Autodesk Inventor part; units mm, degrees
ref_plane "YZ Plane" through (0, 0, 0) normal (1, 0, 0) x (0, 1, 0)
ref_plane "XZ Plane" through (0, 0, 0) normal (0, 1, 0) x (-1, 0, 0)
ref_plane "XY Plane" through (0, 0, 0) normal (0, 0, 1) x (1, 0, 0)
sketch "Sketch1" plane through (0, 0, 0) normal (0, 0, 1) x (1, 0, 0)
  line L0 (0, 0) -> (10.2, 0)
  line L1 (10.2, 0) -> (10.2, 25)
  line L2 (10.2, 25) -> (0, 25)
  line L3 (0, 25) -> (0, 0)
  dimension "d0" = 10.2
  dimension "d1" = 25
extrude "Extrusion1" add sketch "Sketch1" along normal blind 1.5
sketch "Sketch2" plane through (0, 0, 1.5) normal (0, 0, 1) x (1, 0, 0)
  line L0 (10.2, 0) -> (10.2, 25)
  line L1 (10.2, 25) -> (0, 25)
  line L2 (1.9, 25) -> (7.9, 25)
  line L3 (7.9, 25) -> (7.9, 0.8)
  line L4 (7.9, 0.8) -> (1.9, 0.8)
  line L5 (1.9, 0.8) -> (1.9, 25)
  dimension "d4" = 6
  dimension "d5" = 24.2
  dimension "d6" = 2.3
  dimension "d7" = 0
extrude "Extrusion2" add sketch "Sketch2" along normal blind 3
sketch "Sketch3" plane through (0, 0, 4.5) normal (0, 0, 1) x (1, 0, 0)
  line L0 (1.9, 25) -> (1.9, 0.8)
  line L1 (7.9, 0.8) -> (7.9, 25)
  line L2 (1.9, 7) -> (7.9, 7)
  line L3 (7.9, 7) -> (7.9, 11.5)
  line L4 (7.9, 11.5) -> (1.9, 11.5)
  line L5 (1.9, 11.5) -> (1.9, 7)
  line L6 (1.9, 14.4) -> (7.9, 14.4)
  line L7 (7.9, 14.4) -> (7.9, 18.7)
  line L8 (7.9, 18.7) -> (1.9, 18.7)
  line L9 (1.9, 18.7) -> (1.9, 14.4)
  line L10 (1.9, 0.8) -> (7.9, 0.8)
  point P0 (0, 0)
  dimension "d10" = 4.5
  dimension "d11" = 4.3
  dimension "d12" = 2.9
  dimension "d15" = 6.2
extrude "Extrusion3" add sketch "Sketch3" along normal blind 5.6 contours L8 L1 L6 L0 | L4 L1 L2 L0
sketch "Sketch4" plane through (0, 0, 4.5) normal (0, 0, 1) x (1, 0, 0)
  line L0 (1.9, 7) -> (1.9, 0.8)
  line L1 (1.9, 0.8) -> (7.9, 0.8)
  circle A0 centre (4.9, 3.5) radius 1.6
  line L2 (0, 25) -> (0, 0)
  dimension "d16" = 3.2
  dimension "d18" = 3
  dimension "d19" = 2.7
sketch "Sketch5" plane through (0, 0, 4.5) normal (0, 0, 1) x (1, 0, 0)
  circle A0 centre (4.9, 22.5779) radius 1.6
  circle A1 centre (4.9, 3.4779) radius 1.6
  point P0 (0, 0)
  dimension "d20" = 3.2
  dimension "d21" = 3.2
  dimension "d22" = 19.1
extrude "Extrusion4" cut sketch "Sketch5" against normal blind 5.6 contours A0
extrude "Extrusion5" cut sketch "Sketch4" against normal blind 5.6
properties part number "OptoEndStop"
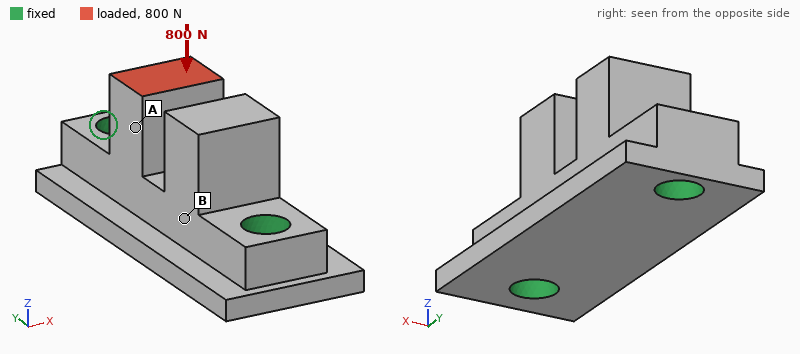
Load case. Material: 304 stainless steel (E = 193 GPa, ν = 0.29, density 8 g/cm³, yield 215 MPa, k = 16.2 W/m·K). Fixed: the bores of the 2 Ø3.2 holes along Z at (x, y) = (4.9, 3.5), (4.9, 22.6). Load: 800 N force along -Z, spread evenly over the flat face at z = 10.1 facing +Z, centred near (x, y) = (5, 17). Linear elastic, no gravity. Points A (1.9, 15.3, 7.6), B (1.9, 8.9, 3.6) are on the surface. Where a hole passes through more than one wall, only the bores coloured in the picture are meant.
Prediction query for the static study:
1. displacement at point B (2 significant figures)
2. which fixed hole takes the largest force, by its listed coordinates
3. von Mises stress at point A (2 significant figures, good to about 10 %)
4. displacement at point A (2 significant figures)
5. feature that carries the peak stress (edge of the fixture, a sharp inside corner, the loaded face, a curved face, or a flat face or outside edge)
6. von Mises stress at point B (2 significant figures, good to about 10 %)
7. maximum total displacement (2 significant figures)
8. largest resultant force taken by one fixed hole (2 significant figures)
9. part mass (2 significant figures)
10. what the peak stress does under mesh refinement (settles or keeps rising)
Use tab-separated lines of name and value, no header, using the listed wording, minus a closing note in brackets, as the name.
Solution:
displacement at point B	1.1 µm
which fixed hole takes the largest force, by its listed coordinates	(4.9, 22.6)
von Mises stress at point A	31 MPa
displacement at point A	3.3 µm
feature that carries the peak stress	edge of the fixture
von Mises stress at point B	13 MPa
maximum total displacement	4.2 µm
largest resultant force taken by one fixed hole	600 N
part mass	8.3 g
what the peak stress does under mesh refinement	keeps rising
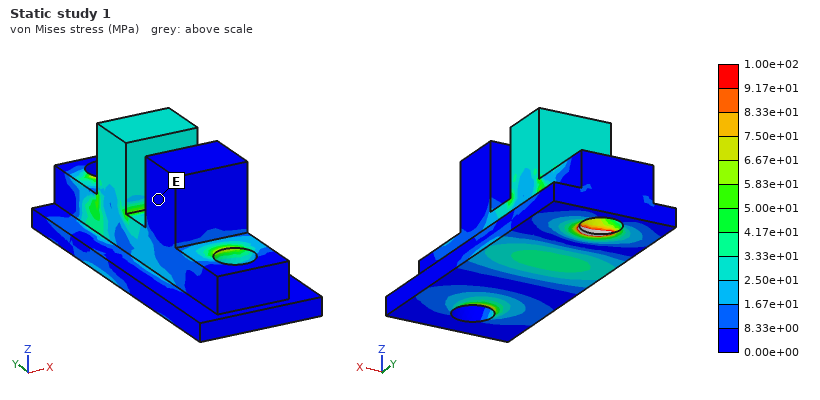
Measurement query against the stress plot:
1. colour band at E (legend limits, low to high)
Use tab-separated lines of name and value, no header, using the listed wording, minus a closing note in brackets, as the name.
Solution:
colour band at E	0.00e+00 to 8.33e+00 MPa
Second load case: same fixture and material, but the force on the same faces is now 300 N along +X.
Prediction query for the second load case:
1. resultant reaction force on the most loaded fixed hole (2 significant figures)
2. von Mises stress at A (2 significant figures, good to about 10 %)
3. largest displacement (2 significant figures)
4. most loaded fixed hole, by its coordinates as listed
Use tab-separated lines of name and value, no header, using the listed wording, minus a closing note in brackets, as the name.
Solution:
resultant reaction force on the most loaded fixed hole	230 N
von Mises stress at A	30 MPa
largest displacement	11 µm
most loaded fixed hole, by its coordinates as listed	(4.9, 22.6)
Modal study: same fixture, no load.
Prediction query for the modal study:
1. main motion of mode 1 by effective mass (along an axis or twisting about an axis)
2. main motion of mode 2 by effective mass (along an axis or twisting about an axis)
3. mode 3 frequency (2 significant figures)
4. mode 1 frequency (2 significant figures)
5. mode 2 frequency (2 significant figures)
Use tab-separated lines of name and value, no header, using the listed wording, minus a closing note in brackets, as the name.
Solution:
main motion of mode 1 by effective mass	along X
main motion of mode 2 by effective mass	along Z
mode 3 frequency	46 kHz
mode 1 frequency	30 kHz
mode 2 frequency	36 kHz
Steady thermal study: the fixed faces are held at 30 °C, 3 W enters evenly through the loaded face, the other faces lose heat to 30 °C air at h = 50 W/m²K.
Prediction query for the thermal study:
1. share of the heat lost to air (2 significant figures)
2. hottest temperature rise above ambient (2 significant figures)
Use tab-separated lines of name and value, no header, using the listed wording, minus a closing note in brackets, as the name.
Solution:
share of the heat lost to air	15 %
hottest temperature rise above ambient	60 K
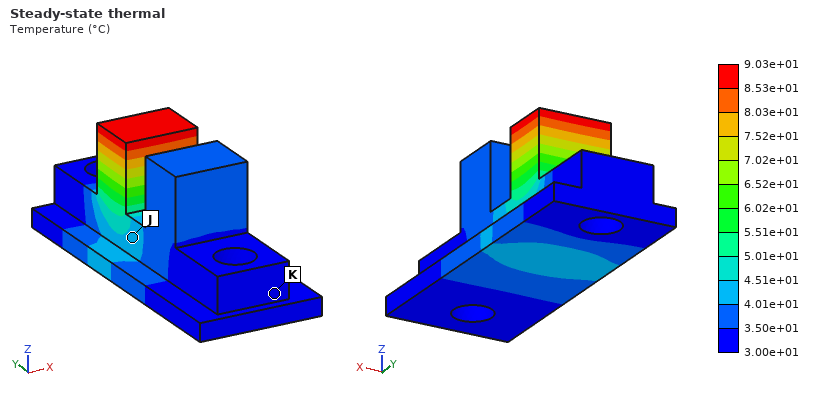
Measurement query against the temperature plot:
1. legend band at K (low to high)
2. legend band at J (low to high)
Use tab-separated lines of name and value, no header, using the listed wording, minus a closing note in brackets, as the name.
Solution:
legend band at K	3.00e+01 to 3.50e+01 °C
legend band at J	4.01e+01 to 4.51e+01 °C
